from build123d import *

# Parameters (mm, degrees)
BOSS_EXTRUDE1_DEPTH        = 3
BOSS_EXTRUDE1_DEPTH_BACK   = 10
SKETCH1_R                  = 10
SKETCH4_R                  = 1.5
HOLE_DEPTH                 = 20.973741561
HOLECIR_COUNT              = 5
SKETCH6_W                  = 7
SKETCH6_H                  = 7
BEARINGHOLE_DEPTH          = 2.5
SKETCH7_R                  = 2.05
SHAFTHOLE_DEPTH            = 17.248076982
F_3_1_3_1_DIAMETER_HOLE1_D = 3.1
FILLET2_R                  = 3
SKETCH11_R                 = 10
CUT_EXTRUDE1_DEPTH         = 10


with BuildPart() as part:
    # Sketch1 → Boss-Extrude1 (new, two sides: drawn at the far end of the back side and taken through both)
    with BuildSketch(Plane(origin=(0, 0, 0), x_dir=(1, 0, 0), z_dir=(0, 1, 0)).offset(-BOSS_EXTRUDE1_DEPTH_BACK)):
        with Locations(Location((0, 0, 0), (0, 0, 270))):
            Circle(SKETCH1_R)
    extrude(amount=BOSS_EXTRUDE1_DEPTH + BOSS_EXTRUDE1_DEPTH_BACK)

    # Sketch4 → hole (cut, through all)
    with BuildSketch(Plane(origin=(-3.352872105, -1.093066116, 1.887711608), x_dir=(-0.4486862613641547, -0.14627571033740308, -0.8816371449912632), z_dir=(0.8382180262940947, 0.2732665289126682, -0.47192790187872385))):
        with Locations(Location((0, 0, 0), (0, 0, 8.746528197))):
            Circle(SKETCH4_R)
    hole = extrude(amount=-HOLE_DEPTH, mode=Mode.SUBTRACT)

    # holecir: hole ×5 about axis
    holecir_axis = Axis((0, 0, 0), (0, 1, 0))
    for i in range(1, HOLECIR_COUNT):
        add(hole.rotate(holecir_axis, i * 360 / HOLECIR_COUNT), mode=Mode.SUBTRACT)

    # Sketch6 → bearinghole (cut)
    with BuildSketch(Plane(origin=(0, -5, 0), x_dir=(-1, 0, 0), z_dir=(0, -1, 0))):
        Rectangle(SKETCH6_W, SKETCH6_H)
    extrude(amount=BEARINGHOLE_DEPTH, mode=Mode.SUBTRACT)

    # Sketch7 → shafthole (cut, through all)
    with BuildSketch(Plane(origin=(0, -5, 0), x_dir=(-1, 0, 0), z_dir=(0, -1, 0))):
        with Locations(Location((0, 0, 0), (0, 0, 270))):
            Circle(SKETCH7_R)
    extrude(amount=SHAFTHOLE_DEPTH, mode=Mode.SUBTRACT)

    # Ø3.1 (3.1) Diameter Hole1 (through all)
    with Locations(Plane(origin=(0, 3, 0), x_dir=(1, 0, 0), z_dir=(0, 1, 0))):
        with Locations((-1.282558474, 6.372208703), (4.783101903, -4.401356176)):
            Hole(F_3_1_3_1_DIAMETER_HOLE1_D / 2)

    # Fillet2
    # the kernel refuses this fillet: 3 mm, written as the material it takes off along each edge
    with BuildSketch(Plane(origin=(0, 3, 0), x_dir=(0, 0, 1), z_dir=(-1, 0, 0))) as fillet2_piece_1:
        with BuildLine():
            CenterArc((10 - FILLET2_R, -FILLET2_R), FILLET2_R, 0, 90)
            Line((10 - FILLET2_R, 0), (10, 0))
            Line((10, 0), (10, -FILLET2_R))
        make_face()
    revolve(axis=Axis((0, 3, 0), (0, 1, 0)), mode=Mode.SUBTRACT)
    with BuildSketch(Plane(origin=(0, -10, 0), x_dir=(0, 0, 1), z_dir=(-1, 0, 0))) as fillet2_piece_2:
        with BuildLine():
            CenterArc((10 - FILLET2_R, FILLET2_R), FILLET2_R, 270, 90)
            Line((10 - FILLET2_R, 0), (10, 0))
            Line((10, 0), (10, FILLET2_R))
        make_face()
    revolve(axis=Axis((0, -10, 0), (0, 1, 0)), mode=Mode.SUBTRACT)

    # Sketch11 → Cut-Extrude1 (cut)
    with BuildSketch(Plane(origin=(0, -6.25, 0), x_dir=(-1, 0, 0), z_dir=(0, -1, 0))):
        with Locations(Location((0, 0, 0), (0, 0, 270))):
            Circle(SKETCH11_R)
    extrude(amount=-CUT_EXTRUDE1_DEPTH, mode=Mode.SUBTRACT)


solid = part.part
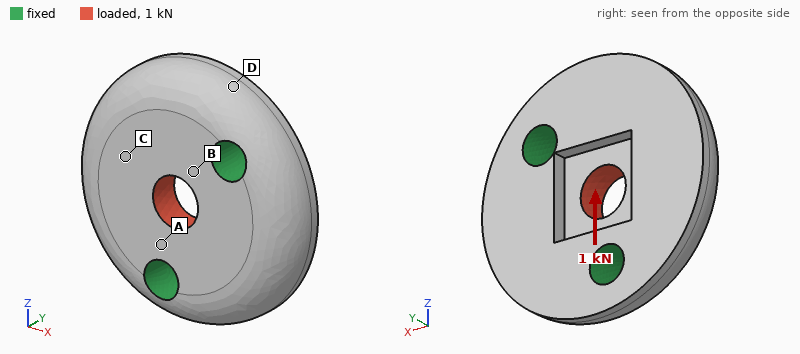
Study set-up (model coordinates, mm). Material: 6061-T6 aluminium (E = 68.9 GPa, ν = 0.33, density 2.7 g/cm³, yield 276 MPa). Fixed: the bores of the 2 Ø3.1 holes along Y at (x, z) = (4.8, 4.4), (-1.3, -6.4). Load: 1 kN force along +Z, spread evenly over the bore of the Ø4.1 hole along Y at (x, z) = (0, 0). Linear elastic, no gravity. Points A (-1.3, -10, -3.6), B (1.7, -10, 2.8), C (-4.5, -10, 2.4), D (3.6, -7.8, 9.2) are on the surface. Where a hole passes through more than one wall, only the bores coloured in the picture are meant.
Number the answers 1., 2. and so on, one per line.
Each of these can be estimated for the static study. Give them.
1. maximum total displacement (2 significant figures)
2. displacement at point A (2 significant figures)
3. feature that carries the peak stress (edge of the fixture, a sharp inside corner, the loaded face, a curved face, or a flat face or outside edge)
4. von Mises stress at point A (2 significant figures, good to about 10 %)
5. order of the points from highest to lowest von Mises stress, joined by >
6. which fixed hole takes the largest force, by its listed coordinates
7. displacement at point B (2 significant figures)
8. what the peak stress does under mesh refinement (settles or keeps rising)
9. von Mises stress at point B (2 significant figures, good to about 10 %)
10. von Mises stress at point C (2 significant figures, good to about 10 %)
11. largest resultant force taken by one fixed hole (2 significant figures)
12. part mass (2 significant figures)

1. 3.6 µm
2. 0.93 µm
3. edge of the fixture
4. 43 MPa
5. A > B > C > D
6. (-1.3, -6.4)
7. 1.8 µm
8. keeps rising
9. 31 MPa
10. 13 MPa
11. 560 N
12. 2.5 g
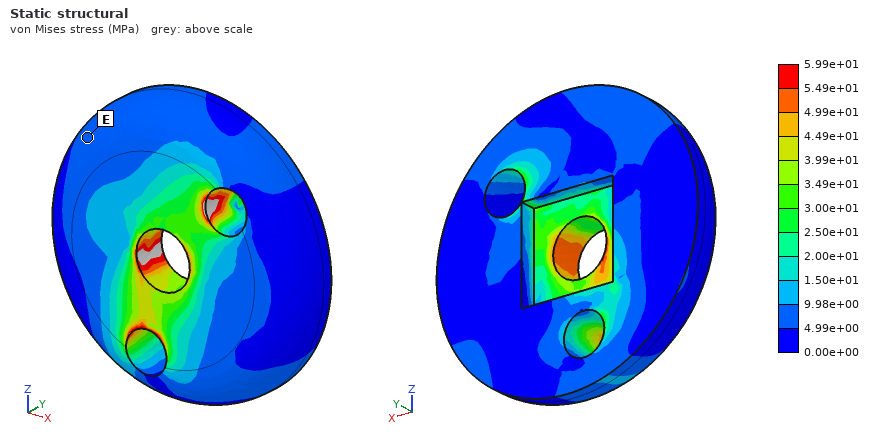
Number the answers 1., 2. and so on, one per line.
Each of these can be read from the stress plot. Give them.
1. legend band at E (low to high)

1. 4.99e+00 to 9.98e+00 MPa
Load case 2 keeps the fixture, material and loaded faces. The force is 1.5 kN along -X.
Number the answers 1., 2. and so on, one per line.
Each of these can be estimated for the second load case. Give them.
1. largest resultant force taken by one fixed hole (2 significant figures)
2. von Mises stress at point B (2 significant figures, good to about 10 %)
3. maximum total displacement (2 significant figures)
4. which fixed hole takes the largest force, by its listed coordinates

1. 840 N
2. 58 MPa
3. 5.6 µm
4. (4.8, 4.4)
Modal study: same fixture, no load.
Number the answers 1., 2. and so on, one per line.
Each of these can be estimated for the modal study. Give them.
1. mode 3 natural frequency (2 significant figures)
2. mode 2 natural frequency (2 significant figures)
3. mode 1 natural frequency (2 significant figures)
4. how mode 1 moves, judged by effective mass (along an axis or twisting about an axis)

1. 53 kHz
2. 53 kHz
3. 25 kHz
4. along Y
